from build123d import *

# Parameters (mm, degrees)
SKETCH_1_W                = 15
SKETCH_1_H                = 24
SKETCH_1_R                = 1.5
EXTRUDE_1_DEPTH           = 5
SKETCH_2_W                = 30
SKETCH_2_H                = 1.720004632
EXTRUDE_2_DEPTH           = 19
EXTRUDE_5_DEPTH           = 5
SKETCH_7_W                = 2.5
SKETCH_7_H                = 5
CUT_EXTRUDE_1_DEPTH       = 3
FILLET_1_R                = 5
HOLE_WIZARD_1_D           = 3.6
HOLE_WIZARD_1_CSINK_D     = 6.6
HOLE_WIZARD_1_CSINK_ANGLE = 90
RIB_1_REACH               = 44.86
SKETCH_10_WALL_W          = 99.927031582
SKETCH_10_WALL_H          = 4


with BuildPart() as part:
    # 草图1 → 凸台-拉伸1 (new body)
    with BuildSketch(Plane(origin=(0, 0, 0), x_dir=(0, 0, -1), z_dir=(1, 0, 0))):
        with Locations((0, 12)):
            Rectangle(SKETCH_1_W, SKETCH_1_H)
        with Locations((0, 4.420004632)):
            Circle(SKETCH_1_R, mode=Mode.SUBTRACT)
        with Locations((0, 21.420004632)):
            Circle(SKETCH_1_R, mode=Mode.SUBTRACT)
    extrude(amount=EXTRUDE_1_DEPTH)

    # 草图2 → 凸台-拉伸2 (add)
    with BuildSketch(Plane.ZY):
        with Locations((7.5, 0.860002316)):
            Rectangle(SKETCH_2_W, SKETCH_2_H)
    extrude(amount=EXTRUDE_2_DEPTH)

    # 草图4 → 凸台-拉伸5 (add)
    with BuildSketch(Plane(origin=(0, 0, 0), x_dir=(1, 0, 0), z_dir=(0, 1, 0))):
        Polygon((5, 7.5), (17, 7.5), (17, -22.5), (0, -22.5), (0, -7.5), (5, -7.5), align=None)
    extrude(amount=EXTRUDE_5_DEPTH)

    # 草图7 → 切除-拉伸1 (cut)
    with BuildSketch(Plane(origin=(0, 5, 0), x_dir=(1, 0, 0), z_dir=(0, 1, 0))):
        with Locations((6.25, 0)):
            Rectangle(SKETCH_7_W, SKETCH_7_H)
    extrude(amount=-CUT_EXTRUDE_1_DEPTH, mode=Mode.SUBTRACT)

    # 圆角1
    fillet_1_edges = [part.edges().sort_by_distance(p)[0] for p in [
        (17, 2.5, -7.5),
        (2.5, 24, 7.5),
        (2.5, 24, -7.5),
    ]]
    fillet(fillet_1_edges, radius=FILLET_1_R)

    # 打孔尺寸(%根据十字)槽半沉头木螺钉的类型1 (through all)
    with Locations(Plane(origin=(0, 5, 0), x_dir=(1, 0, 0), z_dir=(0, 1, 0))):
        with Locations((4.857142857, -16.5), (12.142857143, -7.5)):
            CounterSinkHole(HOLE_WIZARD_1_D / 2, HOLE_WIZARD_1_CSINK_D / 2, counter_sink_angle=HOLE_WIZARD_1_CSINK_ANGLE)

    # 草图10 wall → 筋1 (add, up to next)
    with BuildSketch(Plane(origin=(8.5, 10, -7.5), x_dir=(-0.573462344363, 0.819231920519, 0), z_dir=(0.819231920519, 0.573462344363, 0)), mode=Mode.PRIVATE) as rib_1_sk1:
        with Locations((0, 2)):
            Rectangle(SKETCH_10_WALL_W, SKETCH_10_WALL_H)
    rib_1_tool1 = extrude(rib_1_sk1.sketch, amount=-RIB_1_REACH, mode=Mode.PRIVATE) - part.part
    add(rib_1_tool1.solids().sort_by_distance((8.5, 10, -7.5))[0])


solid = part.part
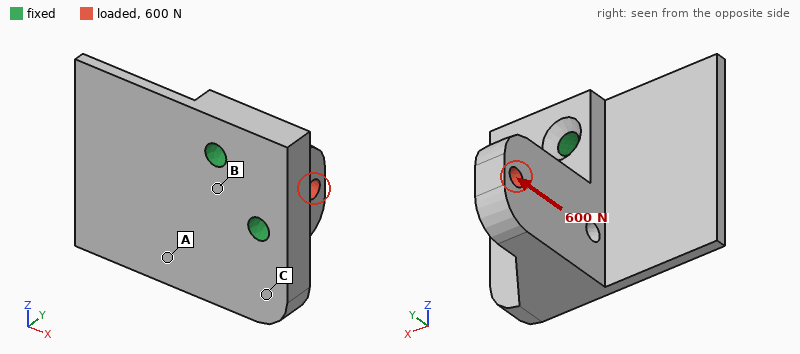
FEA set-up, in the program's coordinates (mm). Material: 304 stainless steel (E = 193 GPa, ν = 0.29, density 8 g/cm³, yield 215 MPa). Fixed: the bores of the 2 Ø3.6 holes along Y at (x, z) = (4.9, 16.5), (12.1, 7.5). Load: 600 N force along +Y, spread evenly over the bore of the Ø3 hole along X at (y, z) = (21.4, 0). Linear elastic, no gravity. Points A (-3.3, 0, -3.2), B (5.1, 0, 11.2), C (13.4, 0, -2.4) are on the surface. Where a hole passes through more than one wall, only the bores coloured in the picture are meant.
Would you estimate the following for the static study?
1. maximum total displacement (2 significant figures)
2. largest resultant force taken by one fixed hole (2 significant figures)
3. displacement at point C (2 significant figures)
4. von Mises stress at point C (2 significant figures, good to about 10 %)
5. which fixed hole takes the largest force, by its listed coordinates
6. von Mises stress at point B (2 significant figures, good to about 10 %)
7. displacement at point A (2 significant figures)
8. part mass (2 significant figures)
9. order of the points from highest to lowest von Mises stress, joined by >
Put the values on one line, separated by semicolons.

38 µm; 510 N; 6.3 µm; 26 MPa; (12.1, 7.5); 50 MPa; 23 µm; 38 g; B > C > A
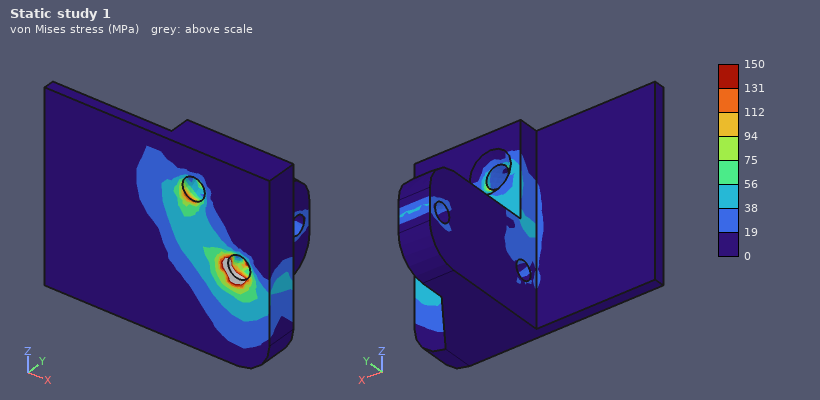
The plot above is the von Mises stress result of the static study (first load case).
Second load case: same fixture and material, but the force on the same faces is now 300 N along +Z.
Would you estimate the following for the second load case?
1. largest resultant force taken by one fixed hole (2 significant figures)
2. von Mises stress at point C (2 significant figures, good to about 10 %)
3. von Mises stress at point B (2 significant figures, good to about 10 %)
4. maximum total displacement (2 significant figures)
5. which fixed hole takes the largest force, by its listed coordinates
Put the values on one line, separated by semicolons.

410 N; 26 MPa; 26 MPa; 36 µm; (4.9, 16.5)
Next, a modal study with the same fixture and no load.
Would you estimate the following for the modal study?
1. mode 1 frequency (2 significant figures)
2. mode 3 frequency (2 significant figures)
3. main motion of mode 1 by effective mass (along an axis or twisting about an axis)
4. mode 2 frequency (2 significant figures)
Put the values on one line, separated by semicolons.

3200 Hz; 6700 Hz; along Y; 4800 Hz
